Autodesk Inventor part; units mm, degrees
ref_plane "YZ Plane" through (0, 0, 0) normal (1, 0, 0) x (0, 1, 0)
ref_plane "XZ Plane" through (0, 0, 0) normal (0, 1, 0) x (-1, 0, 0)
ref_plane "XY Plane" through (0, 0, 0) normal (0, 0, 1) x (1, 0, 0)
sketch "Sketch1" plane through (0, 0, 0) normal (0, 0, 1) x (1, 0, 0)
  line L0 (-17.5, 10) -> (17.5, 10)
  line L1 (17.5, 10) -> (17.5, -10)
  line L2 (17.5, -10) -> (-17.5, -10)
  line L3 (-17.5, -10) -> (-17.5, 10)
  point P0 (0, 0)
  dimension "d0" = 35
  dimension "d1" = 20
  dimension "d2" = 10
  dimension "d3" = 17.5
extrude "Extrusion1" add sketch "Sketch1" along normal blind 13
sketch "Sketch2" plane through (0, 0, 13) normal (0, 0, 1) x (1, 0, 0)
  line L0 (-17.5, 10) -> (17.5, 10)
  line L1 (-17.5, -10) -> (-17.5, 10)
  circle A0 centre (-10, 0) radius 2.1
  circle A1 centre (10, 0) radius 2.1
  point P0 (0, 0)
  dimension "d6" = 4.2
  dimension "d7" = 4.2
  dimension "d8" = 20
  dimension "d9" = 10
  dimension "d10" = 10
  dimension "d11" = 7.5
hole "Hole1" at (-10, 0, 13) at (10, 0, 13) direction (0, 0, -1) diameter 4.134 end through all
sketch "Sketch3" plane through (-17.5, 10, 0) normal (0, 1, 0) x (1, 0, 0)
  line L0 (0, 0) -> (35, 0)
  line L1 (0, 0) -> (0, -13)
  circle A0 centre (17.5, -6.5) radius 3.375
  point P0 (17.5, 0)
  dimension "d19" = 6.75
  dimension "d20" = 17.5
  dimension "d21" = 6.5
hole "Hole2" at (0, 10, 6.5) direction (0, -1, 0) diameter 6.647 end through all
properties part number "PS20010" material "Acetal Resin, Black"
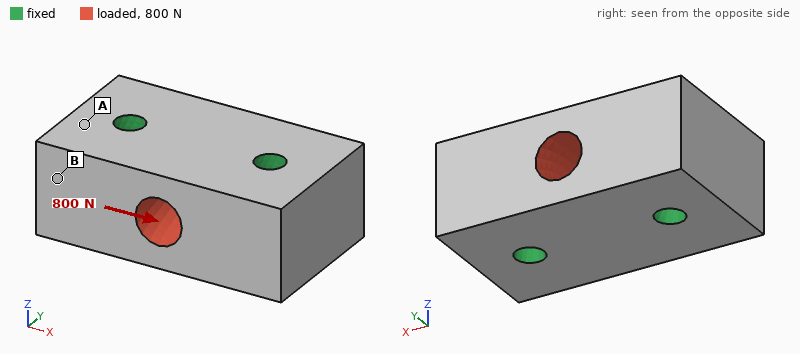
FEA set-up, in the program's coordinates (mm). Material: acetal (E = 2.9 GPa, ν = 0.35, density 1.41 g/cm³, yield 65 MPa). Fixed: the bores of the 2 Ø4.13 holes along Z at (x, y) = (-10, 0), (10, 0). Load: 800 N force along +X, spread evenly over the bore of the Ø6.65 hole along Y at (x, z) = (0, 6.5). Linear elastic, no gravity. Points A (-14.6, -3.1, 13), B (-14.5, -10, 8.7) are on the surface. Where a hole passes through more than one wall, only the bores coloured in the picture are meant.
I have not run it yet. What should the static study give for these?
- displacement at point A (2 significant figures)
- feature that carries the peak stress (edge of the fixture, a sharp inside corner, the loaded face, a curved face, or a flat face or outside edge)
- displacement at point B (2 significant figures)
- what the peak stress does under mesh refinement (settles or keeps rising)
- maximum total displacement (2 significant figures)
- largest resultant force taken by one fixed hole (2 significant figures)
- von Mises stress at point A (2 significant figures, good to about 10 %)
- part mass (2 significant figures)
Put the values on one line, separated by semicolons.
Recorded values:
1.8 µm; edge of the fixture; 5.5 µm; keeps rising; 9.6 µm; 400 N; 1.1 MPa; 11 g
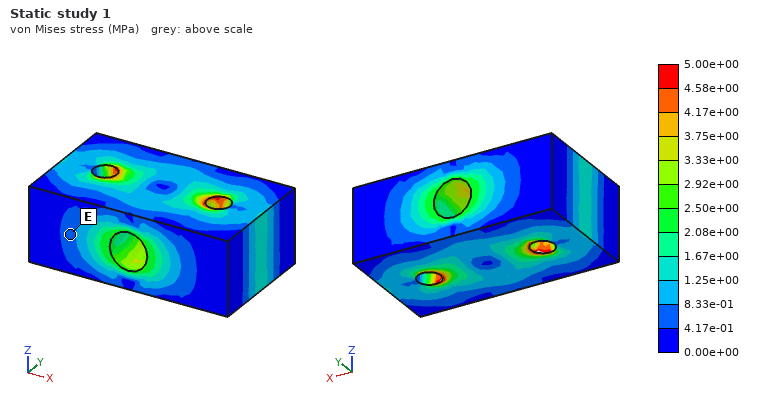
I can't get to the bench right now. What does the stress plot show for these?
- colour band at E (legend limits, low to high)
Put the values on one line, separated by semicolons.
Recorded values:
4.17e-01 to 8.33e-01 MPa
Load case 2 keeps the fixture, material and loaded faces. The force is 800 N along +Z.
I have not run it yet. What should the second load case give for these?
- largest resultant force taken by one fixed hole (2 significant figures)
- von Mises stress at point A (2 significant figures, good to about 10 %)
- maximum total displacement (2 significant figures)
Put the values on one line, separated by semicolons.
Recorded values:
400 N; 1.6 MPa; 26 µm
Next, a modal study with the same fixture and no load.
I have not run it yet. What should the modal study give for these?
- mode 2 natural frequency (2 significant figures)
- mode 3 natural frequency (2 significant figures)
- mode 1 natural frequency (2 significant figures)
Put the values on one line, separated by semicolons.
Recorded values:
15 kHz; 15 kHz; 14 kHz
